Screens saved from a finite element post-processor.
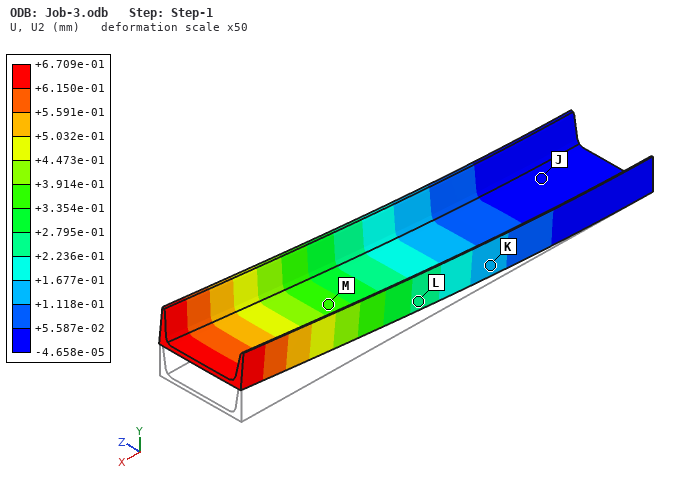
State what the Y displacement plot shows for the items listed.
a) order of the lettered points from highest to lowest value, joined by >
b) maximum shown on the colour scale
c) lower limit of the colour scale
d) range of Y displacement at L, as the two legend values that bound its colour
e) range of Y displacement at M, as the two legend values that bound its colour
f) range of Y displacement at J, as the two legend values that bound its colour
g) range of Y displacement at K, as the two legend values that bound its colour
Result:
M > L > K > J
+6.709e-01 mm
-4.658e-05 mm
+2.236e-01 to +2.795e-01 mm
+3.354e-01 to +3.914e-01 mm
-4.658e-05 to +5.587e-02 mm
+1.118e-01 to +1.677e-01 mm
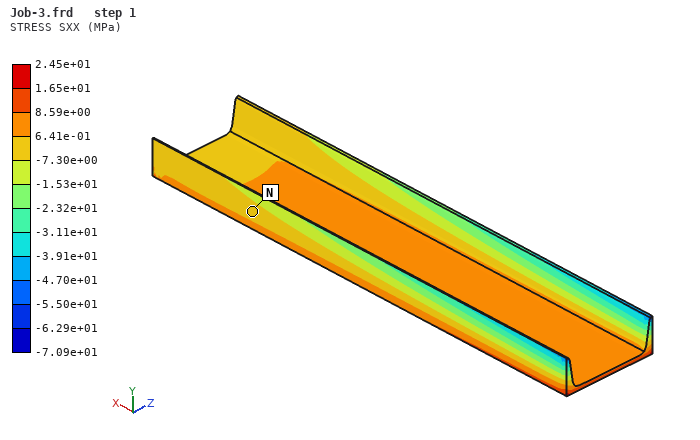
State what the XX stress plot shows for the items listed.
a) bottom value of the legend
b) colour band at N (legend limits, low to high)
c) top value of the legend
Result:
-7.09e+01 MPa
-7.30e+00 to 6.41e-01 MPa
2.45e+01 MPa
